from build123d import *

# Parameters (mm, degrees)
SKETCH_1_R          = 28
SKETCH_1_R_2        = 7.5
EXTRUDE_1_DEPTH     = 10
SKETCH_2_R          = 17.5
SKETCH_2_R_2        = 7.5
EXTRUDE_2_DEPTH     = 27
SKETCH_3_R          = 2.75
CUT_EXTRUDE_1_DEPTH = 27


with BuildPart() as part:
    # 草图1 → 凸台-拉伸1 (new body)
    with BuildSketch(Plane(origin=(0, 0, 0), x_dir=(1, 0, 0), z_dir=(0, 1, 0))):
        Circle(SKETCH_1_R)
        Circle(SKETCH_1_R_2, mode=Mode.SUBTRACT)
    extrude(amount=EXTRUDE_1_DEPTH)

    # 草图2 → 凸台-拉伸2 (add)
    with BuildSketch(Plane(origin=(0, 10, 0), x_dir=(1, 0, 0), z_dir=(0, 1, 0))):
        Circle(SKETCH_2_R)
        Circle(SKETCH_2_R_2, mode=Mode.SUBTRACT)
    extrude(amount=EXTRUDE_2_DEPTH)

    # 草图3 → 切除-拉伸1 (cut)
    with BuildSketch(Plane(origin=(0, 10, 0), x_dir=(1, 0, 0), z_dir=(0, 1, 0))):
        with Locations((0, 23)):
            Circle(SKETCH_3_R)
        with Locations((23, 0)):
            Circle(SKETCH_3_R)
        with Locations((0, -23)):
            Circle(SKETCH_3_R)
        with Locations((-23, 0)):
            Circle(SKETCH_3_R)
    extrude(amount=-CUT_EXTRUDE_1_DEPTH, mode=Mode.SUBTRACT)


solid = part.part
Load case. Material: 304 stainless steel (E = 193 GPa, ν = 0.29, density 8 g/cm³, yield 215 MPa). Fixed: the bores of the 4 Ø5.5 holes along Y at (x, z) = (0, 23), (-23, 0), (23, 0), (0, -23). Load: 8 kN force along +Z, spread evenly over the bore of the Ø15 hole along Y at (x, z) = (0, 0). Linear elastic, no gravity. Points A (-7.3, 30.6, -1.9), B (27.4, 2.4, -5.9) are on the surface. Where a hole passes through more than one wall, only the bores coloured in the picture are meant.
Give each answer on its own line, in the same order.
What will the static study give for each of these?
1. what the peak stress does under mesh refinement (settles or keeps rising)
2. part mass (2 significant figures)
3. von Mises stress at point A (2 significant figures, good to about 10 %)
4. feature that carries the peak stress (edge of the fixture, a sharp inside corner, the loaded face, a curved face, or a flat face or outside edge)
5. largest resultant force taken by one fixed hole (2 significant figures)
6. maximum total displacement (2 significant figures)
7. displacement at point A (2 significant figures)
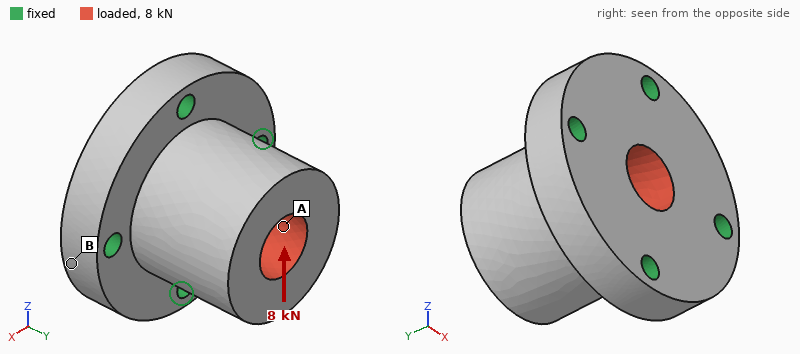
keeps rising
340 g
13 MPa
edge of the fixture
3.5 kN
7.4 µm
5.8 µm
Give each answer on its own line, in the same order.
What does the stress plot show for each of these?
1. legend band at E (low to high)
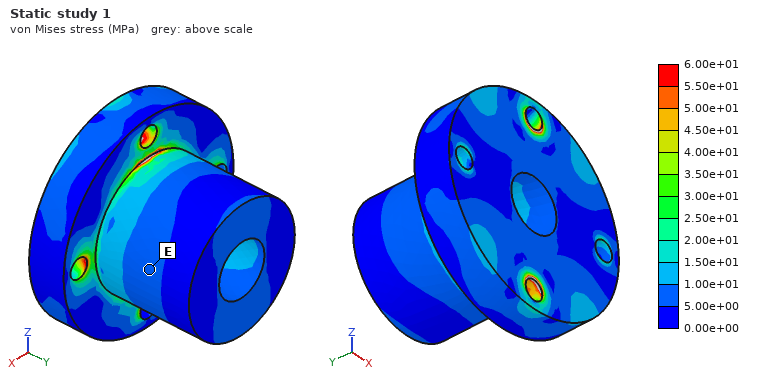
5.00e+00 to 1.00e+01 MPa
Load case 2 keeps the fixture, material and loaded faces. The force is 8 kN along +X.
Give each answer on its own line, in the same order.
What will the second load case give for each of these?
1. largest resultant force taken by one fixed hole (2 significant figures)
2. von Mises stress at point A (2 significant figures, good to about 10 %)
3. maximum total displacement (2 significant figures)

3.5 kN
6.4 MPa
7.4 µm
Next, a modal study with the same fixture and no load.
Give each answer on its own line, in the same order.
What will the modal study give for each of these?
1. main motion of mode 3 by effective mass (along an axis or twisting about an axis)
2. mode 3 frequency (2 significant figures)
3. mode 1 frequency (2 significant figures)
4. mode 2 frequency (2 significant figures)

along Y
20 kHz
13 kHz
13 kHz
